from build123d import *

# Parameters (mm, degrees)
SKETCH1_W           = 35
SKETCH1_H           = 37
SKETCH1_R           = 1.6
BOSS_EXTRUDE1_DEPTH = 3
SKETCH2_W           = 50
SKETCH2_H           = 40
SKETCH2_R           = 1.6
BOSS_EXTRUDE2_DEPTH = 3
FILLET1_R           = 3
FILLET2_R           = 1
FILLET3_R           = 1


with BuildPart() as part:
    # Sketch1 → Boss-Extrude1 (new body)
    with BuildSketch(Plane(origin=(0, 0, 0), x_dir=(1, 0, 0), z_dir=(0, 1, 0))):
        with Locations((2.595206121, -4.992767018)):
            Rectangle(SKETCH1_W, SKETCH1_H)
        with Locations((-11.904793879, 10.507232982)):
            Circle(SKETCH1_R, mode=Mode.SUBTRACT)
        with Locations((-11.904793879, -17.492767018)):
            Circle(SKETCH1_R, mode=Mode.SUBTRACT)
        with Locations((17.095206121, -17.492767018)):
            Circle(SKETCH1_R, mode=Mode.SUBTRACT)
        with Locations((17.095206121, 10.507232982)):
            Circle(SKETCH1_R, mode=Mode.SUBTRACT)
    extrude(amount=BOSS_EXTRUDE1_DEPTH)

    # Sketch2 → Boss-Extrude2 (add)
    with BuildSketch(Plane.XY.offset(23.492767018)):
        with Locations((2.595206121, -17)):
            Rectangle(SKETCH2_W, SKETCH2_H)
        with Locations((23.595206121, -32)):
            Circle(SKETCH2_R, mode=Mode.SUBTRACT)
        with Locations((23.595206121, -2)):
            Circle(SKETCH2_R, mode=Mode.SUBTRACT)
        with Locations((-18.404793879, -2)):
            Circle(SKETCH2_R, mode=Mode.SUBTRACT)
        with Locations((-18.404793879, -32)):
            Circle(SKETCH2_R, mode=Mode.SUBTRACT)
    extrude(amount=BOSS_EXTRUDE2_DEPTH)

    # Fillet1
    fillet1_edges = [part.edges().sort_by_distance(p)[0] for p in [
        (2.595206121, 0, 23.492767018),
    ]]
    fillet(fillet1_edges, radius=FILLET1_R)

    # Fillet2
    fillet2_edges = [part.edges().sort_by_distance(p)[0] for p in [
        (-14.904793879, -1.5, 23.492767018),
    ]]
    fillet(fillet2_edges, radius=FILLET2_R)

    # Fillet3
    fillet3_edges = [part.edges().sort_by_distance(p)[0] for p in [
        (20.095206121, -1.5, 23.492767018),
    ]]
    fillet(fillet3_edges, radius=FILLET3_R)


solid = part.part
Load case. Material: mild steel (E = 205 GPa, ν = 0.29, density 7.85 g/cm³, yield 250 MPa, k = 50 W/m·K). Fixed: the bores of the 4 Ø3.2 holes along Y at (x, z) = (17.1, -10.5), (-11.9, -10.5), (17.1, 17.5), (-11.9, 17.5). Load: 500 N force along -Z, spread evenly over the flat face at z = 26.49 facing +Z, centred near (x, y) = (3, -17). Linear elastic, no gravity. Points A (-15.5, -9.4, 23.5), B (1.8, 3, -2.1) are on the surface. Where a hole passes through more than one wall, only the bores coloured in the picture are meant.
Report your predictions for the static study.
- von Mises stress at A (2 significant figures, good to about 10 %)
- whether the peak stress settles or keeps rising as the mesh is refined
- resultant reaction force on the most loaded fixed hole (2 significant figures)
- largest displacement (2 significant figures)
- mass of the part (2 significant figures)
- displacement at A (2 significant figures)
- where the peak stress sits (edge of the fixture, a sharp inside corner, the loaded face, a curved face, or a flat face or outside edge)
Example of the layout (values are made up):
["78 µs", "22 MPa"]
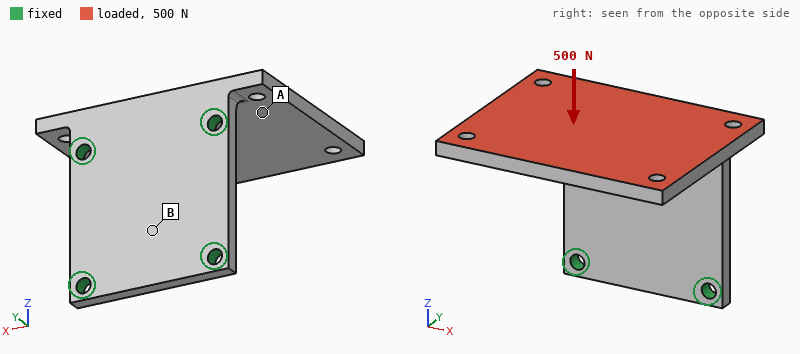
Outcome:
["50 MPa", "keeps rising", "200 N", "0.26 mm", "77 g", "0.053 mm", "edge of the fixture"]
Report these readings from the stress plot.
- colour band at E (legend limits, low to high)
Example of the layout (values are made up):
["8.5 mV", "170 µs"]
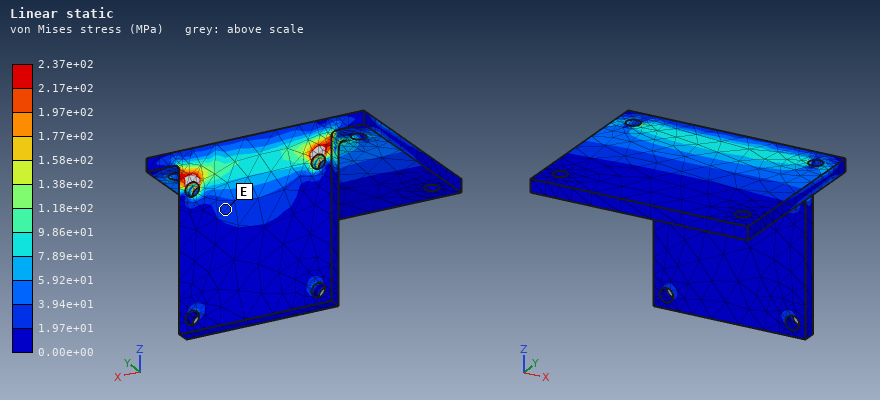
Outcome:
["1.97e+01 to 3.94e+01 MPa"]
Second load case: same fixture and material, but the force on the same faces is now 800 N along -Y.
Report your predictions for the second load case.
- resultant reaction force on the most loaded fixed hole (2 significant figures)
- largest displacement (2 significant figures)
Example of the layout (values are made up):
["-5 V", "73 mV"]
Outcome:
["430 N", "95 µm"]
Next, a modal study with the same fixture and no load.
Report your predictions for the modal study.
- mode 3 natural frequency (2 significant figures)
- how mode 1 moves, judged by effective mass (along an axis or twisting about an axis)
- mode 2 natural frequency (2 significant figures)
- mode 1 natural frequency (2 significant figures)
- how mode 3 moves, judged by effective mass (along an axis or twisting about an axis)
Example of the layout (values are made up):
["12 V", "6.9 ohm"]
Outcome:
["5200 Hz", "along Z", "2800 Hz", "1300 Hz", "along X"]
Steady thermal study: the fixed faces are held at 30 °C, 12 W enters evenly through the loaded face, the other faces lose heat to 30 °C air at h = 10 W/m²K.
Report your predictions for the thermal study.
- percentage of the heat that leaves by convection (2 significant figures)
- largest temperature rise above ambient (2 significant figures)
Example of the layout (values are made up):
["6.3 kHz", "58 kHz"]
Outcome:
["8.4 %", "45 K"]
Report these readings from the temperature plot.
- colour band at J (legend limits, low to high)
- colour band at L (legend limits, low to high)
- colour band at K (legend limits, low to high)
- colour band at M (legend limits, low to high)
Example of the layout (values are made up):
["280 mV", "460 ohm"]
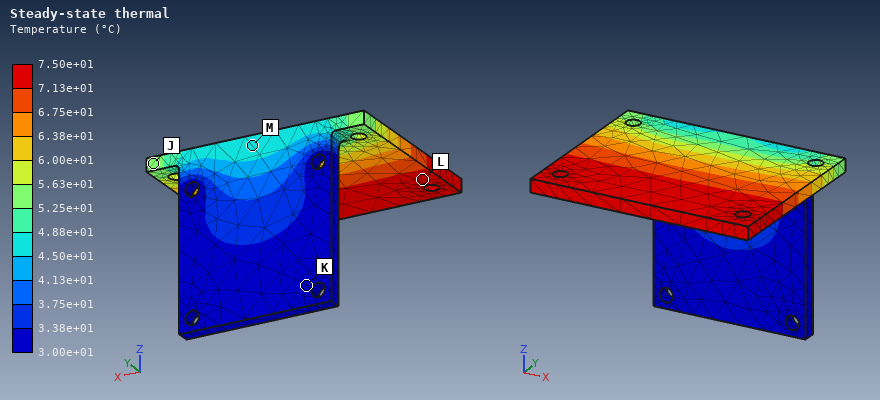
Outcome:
["5.25e+01 to 5.63e+01 °C", "7.13e+01 to 7.50e+01 °C", "3.00e+01 to 3.38e+01 °C", "4.50e+01 to 4.88e+01 °C"]
